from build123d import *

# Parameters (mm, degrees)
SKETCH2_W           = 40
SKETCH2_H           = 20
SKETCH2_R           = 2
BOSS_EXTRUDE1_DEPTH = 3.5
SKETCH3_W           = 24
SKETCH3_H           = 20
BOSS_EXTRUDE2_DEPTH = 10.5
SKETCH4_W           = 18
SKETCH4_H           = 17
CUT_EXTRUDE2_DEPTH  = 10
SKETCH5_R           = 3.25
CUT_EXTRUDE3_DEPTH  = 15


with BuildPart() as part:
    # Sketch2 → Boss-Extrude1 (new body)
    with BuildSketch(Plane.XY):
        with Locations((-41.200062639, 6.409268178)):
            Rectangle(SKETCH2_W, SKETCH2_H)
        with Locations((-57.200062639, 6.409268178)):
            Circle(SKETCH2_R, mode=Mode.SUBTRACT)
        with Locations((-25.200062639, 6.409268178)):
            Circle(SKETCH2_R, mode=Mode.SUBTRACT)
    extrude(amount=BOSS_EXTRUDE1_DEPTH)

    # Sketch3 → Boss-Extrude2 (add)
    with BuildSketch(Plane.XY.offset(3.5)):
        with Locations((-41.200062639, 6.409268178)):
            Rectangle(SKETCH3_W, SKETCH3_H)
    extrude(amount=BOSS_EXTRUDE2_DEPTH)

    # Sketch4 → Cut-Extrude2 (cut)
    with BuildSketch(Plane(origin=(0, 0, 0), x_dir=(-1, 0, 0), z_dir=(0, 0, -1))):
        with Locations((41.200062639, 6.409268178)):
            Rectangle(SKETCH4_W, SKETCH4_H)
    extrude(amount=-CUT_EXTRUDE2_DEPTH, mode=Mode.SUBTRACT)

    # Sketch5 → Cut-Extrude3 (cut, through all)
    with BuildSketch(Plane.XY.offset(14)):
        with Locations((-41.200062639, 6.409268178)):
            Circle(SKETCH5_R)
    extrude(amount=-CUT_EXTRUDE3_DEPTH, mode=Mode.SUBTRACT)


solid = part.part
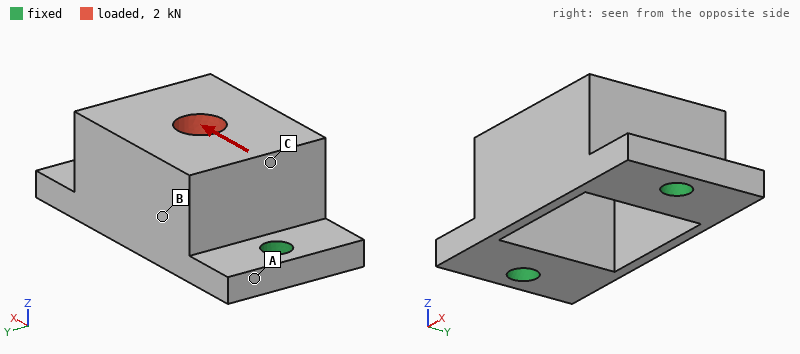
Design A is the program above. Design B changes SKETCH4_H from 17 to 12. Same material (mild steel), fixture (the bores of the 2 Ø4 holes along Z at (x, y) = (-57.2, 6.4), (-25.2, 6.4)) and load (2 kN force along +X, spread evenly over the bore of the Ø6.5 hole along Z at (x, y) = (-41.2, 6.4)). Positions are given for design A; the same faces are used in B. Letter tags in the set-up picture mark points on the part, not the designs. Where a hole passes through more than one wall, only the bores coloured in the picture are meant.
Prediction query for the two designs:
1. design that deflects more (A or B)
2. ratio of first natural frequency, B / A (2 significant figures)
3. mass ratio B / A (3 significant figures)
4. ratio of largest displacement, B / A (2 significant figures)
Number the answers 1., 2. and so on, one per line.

1. A
2. 0.94
3. 1.20
4. 0.75
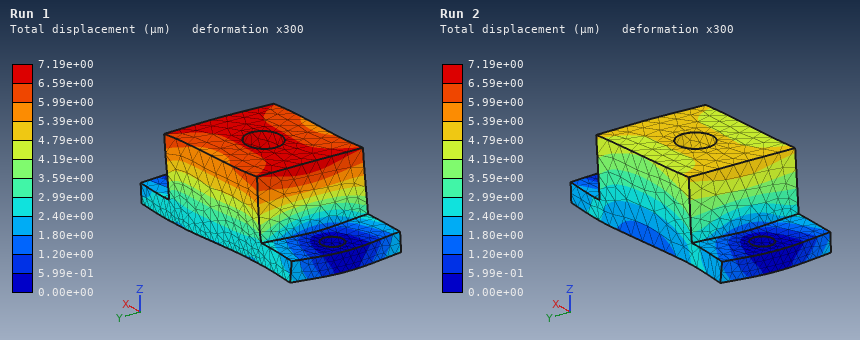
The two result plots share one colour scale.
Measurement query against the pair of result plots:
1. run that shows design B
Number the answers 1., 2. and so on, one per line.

1. Run 2
